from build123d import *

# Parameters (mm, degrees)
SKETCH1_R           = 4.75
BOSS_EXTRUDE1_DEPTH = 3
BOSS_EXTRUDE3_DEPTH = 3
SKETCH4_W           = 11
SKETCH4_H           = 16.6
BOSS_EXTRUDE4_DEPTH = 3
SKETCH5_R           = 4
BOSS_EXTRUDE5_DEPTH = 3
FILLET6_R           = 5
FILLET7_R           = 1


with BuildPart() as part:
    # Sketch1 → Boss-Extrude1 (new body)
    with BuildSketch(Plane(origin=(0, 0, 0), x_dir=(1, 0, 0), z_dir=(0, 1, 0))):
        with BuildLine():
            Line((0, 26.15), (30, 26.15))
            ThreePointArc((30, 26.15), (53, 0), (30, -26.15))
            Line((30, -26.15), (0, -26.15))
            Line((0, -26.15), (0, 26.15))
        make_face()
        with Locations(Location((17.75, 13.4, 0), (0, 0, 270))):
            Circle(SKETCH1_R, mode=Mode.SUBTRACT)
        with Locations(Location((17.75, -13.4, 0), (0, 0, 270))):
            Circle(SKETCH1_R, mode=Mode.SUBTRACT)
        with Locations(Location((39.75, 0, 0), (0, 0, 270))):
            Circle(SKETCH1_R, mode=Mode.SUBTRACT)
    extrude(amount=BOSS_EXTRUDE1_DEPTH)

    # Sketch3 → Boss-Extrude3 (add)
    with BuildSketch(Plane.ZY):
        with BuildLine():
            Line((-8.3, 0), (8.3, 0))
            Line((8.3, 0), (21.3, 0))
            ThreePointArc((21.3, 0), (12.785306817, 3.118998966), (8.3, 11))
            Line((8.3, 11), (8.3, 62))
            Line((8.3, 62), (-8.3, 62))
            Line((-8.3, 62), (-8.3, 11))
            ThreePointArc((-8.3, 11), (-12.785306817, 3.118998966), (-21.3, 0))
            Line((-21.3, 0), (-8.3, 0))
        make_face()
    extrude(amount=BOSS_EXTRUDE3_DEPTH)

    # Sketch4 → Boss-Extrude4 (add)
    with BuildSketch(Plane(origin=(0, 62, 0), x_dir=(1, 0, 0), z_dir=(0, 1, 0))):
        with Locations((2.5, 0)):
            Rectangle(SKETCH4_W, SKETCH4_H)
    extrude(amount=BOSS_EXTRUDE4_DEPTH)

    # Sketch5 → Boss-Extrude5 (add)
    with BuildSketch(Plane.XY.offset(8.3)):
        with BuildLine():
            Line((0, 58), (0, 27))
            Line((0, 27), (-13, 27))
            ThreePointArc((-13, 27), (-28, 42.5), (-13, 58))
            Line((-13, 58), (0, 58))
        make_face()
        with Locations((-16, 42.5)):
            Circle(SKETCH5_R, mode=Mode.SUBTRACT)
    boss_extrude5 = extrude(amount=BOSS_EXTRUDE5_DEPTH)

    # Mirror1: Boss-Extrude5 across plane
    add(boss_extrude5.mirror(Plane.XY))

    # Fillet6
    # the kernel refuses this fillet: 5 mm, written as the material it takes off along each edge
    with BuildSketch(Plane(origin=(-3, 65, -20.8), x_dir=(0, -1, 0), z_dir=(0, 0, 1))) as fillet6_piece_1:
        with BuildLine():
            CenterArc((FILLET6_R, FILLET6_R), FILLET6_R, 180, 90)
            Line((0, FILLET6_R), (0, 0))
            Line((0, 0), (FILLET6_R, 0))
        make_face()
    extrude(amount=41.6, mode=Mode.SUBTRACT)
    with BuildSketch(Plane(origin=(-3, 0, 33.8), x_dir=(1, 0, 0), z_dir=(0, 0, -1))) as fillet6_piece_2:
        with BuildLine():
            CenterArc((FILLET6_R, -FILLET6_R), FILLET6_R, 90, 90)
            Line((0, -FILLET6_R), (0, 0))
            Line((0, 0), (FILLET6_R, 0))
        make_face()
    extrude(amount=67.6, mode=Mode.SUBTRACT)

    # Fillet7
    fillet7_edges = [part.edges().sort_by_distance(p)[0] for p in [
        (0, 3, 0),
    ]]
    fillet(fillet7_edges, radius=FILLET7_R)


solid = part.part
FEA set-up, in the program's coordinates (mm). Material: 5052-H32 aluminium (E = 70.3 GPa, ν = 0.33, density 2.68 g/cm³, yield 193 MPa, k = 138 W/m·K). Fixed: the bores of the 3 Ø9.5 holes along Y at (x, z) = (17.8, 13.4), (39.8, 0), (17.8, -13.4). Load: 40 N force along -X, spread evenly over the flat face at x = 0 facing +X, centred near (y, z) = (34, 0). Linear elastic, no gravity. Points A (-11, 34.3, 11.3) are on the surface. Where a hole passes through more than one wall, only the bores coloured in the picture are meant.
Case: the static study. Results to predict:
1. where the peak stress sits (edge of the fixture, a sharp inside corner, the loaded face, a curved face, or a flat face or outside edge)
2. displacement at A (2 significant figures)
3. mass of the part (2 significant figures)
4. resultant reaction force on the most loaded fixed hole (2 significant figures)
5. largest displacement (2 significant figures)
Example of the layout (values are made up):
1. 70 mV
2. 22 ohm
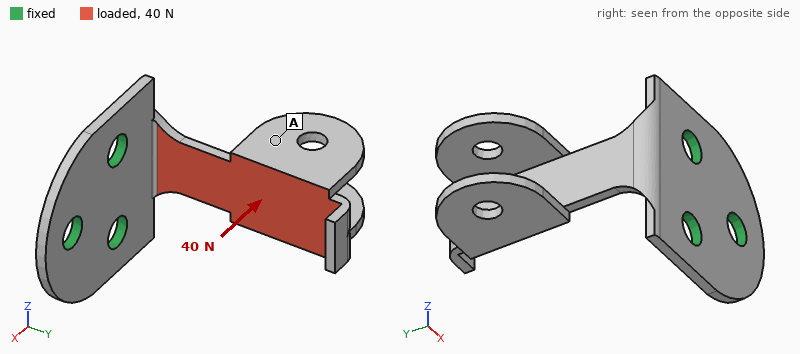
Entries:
1. a curved face
2. 0.30 mm
3. 39 g
4. 20 N
5. 0.63 mm
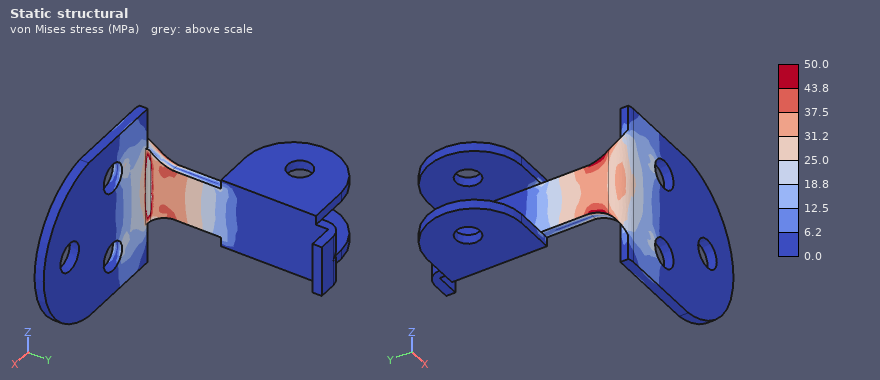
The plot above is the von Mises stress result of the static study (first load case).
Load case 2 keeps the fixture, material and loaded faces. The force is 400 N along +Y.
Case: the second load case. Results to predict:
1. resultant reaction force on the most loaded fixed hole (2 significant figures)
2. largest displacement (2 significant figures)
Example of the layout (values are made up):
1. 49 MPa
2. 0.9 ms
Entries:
1. 210 N
2. 0.14 mm
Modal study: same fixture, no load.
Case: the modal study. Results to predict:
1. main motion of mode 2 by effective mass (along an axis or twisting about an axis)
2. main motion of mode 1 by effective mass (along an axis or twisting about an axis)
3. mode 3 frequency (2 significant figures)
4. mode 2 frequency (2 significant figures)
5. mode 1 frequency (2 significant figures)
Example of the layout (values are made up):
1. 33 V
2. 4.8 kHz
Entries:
1. along Z
2. along X
3. 1100 Hz
4. 840 Hz
5. 300 Hz
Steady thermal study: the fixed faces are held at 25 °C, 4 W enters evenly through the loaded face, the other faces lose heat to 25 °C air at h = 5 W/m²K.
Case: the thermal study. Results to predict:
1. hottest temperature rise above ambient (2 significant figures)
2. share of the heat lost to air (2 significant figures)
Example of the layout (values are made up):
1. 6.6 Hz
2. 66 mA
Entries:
1. 18 K
2. 10.0 %
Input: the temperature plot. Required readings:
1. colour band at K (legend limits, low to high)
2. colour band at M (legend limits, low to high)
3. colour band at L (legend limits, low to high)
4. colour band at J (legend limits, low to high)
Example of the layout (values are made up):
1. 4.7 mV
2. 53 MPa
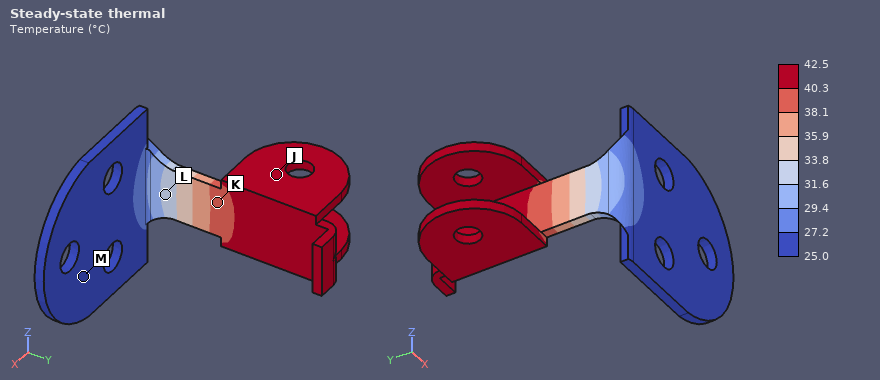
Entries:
1. 38.1 to 40.3 °C
2. 25.0 to 27.2 °C
3. 31.6 to 33.8 °C
4. 40.3 to 42.5 °C
